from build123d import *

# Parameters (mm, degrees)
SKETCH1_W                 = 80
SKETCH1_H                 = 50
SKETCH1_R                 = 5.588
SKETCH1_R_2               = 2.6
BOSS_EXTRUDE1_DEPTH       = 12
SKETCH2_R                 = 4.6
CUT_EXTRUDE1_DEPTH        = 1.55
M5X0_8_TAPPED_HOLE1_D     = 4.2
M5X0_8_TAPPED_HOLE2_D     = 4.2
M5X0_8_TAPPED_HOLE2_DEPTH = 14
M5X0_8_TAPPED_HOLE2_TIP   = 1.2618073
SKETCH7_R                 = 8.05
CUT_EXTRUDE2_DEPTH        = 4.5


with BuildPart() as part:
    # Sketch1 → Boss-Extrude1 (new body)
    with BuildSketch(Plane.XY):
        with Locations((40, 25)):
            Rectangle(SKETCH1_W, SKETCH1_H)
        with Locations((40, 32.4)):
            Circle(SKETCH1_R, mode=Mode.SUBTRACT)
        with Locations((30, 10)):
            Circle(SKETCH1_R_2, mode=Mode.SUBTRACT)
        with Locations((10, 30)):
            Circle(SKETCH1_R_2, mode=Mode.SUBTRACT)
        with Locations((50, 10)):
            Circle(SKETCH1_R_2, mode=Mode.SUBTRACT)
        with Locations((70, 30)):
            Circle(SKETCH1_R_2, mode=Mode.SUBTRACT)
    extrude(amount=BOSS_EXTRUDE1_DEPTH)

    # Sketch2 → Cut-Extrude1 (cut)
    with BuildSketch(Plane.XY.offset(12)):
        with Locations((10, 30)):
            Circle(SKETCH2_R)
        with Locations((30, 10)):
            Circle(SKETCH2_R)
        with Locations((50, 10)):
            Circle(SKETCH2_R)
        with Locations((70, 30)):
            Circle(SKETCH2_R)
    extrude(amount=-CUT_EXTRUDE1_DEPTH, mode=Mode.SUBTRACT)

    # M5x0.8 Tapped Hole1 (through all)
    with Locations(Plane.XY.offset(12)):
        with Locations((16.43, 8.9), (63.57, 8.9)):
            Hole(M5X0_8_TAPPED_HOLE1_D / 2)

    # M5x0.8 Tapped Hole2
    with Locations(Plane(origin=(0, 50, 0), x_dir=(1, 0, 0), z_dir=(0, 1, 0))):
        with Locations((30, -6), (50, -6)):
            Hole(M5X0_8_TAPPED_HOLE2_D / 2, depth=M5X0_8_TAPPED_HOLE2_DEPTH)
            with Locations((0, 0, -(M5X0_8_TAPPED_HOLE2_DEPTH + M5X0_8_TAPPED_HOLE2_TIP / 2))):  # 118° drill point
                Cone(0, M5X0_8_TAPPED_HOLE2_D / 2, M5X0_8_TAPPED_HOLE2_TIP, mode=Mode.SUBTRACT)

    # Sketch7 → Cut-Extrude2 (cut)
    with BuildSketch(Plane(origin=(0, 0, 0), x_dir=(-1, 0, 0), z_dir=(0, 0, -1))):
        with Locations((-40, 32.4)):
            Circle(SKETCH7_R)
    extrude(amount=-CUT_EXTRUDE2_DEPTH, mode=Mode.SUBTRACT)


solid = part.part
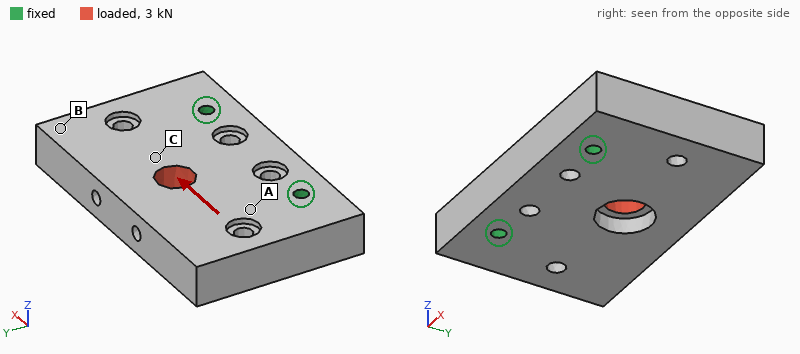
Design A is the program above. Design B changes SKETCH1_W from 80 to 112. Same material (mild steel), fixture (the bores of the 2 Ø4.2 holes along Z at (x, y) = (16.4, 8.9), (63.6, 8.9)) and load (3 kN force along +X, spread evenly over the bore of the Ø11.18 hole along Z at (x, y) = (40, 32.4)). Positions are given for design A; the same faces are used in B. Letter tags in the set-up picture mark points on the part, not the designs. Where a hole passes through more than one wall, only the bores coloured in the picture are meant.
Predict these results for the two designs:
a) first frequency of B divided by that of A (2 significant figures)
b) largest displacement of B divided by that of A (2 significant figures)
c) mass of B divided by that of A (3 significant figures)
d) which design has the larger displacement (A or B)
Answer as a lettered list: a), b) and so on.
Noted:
a) 0.86
b) 1.2
c) 1.43
d) B
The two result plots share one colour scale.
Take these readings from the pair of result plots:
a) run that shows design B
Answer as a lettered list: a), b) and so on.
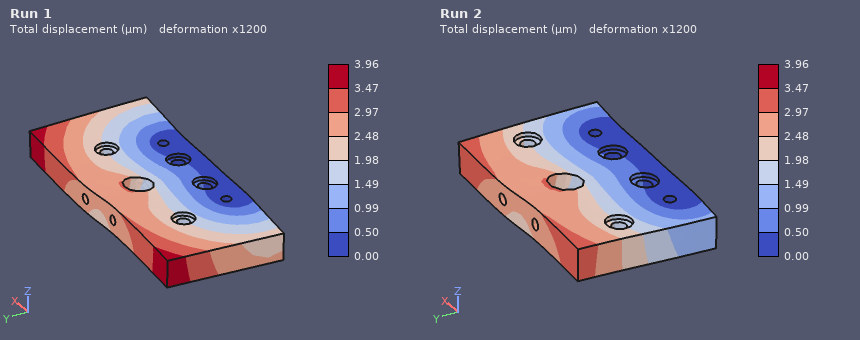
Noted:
a) Run 1
